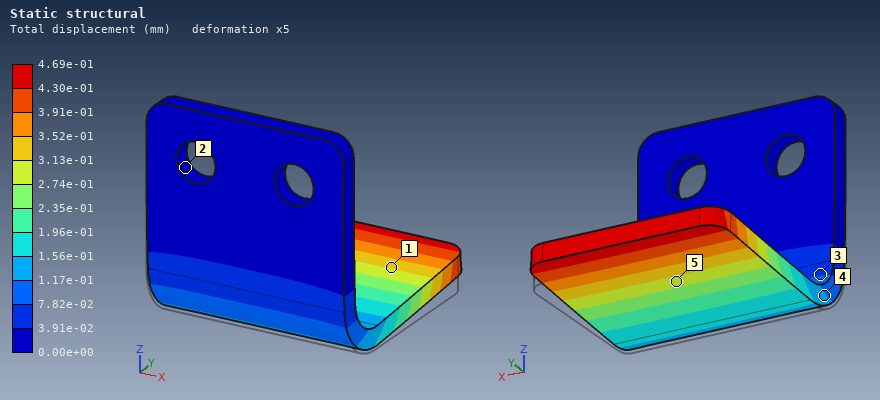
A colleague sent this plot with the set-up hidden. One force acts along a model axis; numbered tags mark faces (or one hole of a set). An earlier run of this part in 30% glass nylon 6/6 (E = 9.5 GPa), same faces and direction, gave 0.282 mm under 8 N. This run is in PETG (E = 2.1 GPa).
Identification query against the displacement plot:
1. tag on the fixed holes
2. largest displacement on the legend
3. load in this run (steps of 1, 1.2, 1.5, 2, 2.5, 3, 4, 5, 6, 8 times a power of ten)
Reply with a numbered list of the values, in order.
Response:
1. 2
2. 4.69e-01 mm
3. 3 N
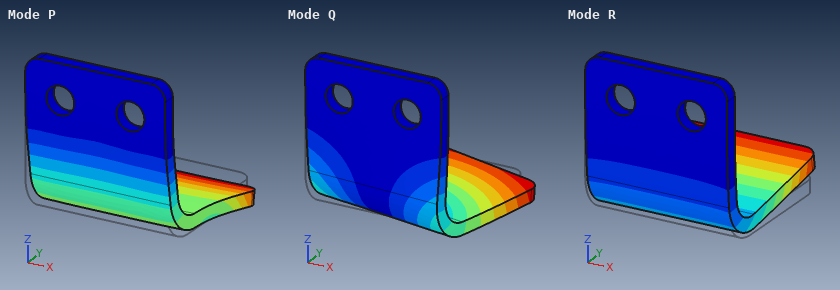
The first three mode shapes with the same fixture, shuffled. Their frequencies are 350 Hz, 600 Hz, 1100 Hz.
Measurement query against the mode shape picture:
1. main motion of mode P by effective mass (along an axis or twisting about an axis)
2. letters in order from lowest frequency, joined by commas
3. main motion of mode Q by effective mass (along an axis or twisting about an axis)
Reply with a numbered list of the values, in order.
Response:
1. along Y
2. R, Q, P
3. along X
